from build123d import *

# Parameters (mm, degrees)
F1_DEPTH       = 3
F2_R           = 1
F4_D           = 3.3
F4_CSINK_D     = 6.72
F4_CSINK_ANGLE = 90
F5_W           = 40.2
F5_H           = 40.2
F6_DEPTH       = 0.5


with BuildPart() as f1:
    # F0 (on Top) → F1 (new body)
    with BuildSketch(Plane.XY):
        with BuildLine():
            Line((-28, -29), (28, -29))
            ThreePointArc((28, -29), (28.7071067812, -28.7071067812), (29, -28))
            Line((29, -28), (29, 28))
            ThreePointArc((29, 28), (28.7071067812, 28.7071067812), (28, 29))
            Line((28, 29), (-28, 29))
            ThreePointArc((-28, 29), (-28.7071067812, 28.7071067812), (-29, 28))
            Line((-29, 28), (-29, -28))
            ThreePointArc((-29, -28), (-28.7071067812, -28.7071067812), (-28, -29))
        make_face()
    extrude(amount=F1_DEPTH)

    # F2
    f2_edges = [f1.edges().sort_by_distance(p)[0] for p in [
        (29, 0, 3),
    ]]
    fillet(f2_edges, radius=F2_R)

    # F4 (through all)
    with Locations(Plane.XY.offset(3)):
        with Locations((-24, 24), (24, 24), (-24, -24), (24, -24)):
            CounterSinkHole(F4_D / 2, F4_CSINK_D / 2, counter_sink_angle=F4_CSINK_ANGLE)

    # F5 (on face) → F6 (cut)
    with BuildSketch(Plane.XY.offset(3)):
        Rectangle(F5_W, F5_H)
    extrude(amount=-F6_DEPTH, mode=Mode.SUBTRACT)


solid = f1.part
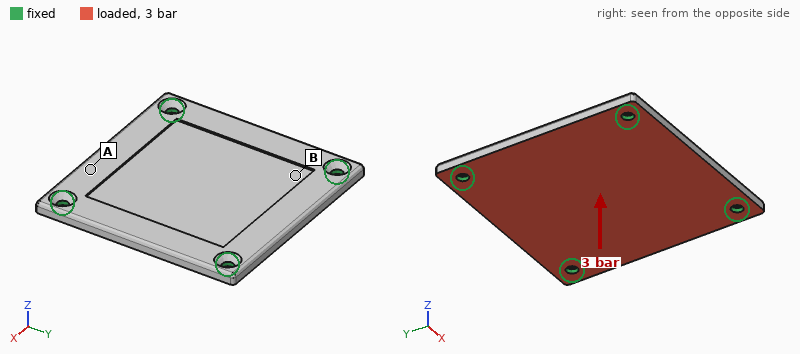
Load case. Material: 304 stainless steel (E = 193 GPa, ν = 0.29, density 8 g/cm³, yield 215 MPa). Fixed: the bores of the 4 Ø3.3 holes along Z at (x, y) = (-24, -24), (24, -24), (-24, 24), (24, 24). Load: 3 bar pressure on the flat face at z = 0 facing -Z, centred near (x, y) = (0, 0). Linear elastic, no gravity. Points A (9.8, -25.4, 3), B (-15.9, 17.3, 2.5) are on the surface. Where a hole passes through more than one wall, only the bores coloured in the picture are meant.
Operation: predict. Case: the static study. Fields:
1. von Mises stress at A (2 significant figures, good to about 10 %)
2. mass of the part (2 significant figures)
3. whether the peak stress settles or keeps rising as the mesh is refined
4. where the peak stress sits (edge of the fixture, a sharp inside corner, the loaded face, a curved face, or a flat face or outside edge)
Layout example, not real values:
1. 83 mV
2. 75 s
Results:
1. 27 MPa
2. 72 g
3. keeps rising
4. edge of the fixture
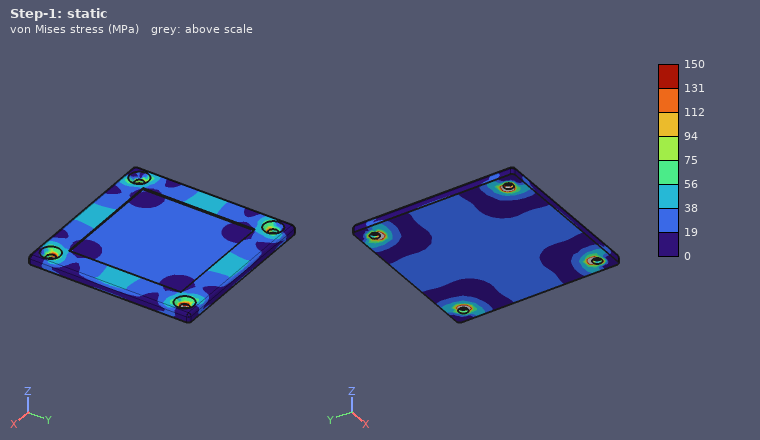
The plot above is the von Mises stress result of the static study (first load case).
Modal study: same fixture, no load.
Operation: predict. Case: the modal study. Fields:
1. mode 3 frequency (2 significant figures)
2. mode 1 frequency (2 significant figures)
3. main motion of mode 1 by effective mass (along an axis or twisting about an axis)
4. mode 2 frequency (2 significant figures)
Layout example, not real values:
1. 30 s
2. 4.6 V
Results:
1. 6000 Hz
2. 3600 Hz
3. along Z
4. 6000 Hz
